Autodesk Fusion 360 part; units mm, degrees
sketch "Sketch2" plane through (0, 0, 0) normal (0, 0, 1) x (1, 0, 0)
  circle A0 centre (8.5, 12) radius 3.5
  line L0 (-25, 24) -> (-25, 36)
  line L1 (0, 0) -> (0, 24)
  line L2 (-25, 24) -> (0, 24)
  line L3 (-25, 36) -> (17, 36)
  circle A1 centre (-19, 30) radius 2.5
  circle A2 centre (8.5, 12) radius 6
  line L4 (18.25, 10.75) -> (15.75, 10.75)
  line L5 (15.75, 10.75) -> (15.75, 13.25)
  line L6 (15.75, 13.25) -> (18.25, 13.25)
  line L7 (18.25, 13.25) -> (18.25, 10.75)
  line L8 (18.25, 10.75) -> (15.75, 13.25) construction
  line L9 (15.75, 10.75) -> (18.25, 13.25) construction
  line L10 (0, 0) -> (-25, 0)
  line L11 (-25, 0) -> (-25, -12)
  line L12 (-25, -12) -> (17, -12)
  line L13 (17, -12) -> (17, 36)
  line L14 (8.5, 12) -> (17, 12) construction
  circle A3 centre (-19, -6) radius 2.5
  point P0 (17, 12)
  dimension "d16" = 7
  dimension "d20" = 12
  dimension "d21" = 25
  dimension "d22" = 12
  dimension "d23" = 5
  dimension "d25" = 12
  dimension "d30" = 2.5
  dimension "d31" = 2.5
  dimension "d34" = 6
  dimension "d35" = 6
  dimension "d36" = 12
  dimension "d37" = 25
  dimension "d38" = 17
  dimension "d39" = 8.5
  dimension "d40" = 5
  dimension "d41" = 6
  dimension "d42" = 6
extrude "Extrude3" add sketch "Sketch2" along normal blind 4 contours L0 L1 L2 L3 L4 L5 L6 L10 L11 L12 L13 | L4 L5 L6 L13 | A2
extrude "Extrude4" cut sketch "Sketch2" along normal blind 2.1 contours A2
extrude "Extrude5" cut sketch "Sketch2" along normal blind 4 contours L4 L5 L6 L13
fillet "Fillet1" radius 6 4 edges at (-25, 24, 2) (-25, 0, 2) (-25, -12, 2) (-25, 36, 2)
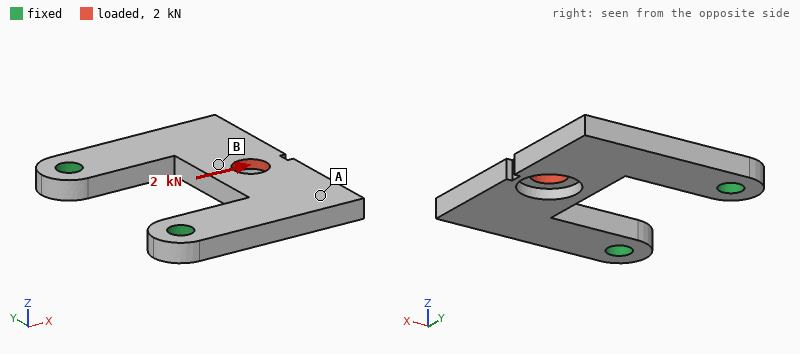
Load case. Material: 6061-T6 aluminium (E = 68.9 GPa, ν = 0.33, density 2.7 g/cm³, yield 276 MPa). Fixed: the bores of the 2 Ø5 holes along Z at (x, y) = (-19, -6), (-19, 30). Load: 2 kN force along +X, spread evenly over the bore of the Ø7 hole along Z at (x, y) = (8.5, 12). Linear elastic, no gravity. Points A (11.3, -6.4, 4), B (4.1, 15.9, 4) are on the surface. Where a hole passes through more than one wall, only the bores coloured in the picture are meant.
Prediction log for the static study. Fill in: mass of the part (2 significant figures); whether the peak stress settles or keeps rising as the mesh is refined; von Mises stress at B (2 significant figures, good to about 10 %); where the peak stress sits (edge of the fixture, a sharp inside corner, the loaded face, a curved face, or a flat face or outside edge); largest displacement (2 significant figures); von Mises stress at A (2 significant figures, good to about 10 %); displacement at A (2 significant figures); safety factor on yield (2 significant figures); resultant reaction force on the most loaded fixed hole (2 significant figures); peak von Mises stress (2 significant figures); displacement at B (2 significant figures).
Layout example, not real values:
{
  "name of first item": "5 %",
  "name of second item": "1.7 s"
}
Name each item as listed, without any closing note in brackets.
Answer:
{
  "mass of the part": "14 g",
  "whether the peak stress settles or keeps rising as the mesh is refined": "settles",
  "von Mises stress at B": "57 MPa",
  "where the peak stress sits": "a flat face or outside edge",
  "largest displacement": "0.15 mm",
  "von Mises stress at A": "15 MPa",
  "displacement at A": "0.095 mm",
  "safety factor on yield": "1.6",
  "resultant reaction force on the most loaded fixed hole": "1.0 kN",
  "peak von Mises stress": "180 MPa",
  "displacement at B": "0.070 mm"
}
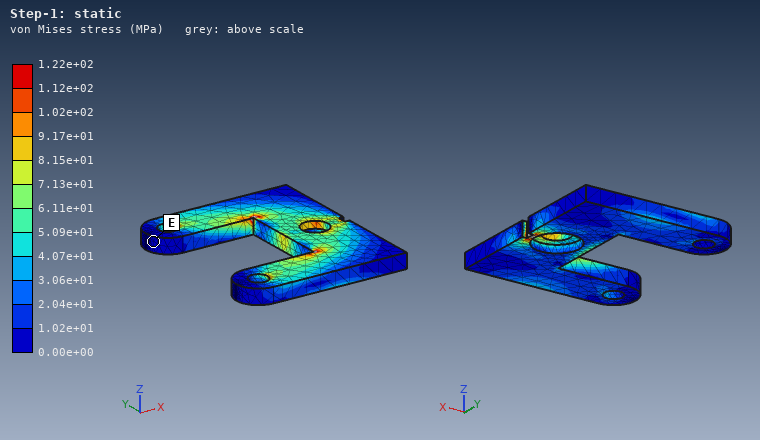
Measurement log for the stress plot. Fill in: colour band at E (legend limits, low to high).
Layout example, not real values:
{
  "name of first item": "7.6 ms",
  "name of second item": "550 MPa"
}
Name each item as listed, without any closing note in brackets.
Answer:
{
  "colour band at E": "0.00e+00 to 1.02e+01 MPa"
}
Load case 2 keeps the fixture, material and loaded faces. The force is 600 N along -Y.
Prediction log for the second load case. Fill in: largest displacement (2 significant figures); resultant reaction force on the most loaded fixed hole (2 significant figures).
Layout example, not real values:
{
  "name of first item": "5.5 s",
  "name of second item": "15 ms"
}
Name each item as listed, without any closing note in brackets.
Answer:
{
  "largest displacement": "29 µm",
  "resultant reaction force on the most loaded fixed hole": "390 N"
}
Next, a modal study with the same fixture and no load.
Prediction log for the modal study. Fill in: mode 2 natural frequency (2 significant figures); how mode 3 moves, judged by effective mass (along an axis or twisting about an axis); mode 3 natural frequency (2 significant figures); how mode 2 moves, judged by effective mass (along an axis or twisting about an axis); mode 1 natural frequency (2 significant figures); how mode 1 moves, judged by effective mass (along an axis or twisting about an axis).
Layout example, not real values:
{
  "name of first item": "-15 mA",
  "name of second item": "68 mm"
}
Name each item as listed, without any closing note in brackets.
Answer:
{
  "mode 2 natural frequency": "4200 Hz",
  "how mode 3 moves, judged by effective mass": "along Y",
  "mode 3 natural frequency": "8500 Hz",
  "how mode 2 moves, judged by effective mass": "twisting about X",
  "mode 1 natural frequency": "2000 Hz",
  "how mode 1 moves, judged by effective mass": "along Z"
}
